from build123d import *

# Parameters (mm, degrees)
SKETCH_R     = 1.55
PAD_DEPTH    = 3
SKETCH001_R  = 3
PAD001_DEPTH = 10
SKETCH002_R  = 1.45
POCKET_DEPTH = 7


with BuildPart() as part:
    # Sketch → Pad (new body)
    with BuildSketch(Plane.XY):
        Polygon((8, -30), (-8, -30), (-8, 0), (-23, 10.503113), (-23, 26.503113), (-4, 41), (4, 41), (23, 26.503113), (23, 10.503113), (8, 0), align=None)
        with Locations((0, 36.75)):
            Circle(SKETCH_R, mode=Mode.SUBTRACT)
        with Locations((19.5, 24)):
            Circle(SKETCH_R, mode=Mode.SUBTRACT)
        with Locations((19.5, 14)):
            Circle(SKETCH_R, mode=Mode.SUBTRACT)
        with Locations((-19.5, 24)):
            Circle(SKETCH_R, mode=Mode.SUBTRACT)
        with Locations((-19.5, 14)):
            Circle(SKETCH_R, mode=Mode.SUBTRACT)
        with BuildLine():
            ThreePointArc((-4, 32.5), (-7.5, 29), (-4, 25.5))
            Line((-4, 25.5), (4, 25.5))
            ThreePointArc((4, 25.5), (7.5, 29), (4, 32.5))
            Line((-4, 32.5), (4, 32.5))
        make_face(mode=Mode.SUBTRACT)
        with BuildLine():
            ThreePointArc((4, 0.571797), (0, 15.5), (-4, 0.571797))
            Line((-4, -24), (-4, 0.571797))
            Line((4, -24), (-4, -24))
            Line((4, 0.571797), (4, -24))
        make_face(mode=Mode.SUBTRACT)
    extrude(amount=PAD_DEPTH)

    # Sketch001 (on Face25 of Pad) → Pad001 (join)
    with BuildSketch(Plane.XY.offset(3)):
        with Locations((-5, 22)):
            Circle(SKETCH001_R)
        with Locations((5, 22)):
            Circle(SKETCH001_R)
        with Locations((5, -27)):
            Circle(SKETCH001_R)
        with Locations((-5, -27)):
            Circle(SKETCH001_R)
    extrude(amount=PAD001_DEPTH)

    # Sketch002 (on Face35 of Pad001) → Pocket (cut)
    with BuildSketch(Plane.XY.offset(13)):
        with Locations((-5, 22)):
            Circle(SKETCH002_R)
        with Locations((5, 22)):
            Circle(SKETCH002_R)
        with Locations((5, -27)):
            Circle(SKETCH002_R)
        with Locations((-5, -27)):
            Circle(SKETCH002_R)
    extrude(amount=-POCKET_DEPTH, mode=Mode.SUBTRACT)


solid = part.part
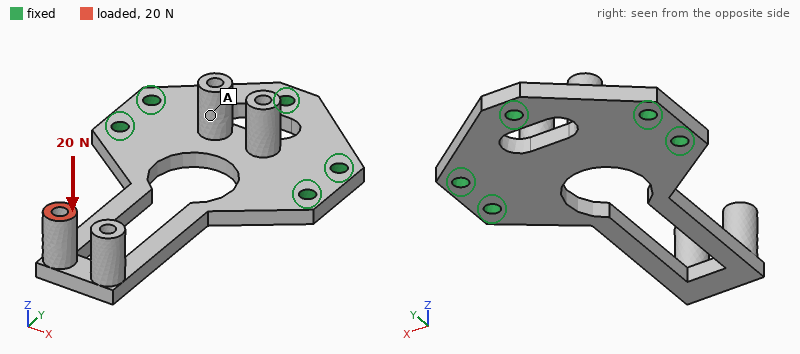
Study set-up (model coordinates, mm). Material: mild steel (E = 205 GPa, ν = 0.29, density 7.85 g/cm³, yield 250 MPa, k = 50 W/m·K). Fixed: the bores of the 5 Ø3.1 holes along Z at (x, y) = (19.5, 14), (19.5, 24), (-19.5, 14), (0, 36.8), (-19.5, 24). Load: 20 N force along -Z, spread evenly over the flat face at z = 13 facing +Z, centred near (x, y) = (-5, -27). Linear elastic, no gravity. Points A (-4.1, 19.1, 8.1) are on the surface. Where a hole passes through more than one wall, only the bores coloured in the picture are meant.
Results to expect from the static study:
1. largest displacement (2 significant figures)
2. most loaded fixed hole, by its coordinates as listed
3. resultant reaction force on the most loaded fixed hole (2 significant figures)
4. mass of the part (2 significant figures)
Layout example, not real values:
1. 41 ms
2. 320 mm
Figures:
1. 0.13 mm
2. (-19.5, 14)
3. 31 N
4. 41 g
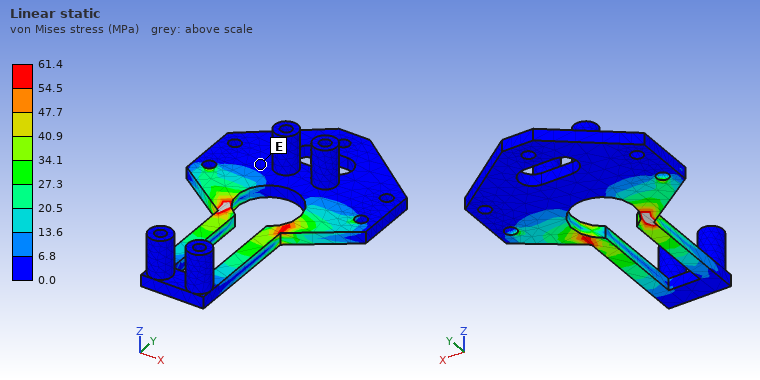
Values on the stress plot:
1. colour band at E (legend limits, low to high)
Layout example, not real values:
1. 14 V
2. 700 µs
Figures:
1. 0.0 to 6.8 MPa
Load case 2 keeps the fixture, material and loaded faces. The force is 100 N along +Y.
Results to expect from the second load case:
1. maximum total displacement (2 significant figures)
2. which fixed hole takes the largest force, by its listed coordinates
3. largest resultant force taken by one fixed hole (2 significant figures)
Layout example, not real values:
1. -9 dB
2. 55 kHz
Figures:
1. 0.30 mm
2. (-19.5, 24)
3. 54 N
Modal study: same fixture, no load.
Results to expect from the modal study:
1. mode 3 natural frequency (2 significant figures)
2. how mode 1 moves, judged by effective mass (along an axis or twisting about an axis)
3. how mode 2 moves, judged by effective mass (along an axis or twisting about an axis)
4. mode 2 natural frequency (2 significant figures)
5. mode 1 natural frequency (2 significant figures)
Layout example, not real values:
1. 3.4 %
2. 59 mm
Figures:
1. 3800 Hz
2. along Z
3. along X
4. 2400 Hz
5. 810 Hz
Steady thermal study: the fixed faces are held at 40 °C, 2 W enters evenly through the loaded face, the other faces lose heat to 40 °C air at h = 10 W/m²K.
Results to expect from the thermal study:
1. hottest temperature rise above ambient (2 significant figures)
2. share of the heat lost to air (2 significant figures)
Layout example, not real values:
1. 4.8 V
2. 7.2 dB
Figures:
1. 67 K
2. 31 %
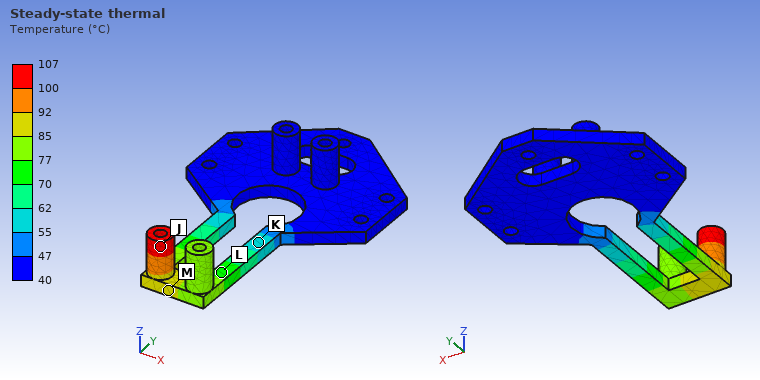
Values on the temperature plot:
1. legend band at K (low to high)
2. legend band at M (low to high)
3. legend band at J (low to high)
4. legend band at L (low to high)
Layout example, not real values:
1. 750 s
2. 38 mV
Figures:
1. 55 to 62 °C
2. 85 to 92 °C
3. 100 to 107 °C
4. 70 to 77 °C
